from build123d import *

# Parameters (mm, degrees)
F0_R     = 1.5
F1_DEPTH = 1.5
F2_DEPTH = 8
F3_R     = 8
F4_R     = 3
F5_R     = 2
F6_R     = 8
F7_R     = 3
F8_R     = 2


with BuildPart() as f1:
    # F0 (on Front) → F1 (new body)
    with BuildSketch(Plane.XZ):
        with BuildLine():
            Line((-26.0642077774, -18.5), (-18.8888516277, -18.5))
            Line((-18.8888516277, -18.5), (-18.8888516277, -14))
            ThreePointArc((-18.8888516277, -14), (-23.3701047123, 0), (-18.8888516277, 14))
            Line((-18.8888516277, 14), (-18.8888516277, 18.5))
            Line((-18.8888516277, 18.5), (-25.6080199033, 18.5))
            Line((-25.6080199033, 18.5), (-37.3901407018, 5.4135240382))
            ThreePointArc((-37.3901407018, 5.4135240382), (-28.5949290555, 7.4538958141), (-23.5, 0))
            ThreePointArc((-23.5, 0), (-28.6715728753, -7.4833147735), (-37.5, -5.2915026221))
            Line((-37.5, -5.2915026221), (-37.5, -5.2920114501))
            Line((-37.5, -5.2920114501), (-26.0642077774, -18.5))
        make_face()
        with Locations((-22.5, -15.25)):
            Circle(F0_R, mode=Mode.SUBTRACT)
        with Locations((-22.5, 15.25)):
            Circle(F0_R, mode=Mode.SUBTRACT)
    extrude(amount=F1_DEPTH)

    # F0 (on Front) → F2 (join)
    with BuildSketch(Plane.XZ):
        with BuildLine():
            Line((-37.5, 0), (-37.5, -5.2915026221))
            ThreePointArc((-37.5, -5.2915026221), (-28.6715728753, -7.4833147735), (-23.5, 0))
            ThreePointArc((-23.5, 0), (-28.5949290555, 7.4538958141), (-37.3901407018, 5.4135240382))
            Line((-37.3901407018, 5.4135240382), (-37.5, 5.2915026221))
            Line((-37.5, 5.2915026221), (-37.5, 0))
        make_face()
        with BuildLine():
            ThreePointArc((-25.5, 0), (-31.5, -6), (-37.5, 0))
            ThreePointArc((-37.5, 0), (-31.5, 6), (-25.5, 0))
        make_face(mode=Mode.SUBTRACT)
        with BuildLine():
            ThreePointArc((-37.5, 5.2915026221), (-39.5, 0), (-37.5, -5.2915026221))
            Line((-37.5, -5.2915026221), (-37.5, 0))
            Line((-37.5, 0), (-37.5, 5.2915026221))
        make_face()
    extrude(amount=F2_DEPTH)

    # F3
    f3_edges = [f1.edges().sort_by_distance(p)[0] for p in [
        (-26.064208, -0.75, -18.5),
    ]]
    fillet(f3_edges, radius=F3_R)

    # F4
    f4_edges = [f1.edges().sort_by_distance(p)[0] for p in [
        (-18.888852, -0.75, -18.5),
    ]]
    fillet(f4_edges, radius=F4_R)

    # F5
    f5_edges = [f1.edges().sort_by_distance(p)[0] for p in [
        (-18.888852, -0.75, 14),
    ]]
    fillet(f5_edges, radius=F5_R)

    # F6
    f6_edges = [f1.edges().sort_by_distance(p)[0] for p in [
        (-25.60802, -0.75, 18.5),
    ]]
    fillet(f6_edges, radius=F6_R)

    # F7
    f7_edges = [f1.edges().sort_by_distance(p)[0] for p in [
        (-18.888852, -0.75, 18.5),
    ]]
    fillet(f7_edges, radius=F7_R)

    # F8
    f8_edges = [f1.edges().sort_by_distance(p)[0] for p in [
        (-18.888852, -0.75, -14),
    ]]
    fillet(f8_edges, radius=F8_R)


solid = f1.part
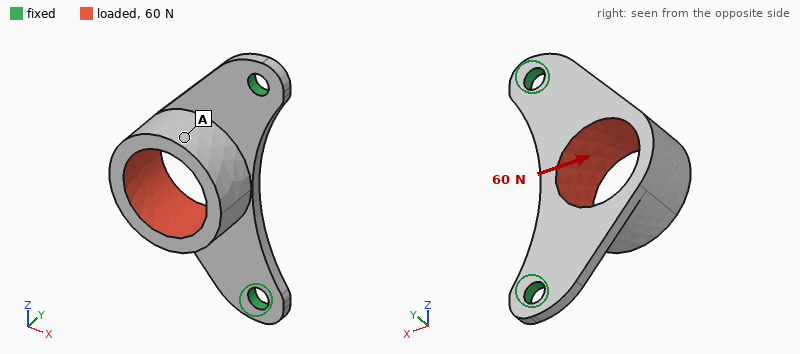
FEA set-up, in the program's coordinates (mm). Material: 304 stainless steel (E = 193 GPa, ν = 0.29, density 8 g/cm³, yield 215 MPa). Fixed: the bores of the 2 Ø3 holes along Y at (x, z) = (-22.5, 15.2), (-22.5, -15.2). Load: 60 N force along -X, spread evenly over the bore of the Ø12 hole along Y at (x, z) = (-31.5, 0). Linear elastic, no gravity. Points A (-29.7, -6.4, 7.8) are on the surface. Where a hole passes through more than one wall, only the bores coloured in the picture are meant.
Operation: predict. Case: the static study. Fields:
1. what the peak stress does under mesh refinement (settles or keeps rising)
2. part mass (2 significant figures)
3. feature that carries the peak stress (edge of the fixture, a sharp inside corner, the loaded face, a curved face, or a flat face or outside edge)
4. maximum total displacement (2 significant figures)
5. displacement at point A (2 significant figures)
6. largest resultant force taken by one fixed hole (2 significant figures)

keeps rising
8.5 g
edge of the fixture
20 µm
8.9 µm
36 N
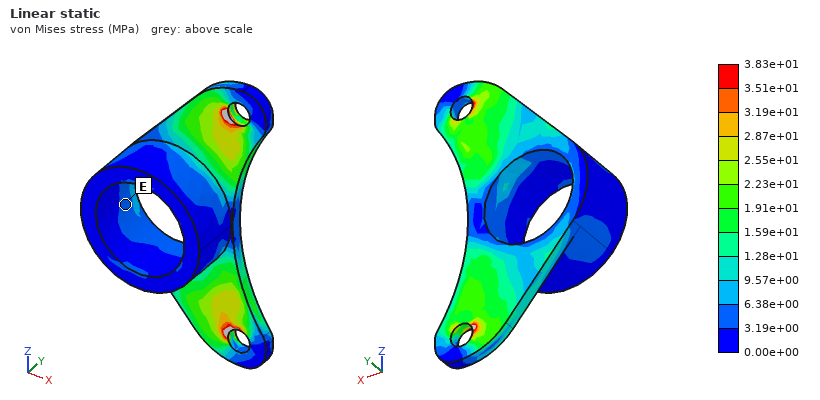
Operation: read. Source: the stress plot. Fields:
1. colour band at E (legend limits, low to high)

3.19e+00 to 6.38e+00 MPa
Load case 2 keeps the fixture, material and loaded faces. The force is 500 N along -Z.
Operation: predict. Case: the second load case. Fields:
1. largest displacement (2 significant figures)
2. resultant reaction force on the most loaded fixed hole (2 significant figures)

15 µm
290 N
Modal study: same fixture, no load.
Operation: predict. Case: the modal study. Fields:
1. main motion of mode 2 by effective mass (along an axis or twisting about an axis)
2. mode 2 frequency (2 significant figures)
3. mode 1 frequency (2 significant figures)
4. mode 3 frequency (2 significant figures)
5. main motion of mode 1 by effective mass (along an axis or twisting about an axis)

along Y
9200 Hz
2900 Hz
11 kHz
along Y
